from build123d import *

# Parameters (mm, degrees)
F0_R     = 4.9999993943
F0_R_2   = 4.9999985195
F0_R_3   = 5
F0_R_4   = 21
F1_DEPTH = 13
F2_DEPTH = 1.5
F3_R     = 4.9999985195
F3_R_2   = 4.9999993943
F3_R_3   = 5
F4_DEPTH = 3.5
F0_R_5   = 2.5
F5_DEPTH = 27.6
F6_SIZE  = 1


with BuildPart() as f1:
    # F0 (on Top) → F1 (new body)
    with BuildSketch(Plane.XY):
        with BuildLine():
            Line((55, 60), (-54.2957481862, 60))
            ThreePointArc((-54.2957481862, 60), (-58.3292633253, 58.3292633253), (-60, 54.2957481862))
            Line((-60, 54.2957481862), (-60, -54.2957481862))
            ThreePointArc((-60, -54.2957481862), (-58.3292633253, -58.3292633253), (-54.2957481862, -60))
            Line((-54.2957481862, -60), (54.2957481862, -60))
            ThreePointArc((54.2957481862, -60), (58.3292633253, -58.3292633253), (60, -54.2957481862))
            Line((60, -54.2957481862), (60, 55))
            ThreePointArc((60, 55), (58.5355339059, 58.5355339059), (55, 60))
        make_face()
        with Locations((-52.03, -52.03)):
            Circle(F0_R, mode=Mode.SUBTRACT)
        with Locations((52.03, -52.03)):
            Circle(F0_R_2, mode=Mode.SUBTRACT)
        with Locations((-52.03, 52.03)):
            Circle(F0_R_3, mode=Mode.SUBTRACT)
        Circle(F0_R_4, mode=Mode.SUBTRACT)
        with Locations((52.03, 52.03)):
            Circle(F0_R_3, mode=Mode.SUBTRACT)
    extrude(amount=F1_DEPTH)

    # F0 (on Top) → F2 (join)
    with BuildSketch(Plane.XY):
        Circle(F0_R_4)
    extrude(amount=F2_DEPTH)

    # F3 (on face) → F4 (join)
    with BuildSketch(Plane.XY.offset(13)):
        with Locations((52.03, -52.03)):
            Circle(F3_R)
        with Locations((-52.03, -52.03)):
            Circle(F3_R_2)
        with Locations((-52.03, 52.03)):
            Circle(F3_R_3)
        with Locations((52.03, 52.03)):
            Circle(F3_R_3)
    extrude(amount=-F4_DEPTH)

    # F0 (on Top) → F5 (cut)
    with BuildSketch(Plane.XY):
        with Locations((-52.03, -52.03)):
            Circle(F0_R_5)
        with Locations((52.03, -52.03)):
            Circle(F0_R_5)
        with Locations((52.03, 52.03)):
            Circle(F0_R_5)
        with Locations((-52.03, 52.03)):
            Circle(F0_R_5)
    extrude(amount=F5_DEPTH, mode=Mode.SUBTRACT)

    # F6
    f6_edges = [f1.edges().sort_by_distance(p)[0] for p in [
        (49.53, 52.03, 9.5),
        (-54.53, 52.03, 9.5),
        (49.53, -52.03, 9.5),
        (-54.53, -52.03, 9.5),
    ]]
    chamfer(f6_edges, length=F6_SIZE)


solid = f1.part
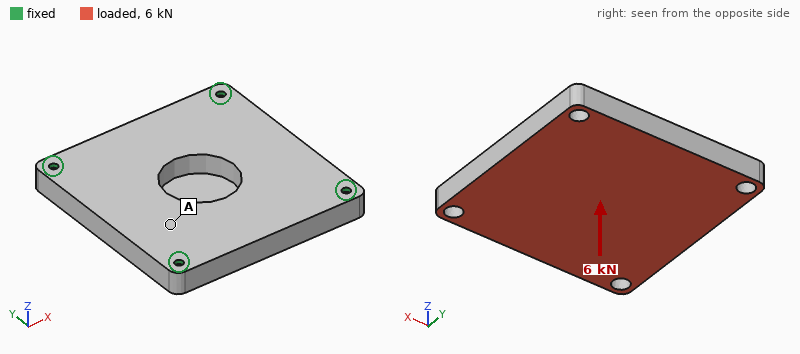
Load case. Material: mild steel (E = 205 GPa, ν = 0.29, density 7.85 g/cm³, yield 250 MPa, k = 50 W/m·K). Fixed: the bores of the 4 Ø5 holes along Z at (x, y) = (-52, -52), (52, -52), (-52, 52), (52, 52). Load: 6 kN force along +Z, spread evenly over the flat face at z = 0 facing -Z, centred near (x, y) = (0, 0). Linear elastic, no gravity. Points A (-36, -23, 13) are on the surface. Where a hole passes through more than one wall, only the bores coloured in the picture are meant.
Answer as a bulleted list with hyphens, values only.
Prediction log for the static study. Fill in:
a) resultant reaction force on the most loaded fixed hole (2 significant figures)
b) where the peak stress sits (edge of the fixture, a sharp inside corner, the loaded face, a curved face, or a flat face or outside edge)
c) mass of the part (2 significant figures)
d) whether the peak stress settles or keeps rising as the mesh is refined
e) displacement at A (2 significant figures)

- 2.7 kN
- edge of the fixture
- 1.3 kg
- keeps rising
- 15 µm
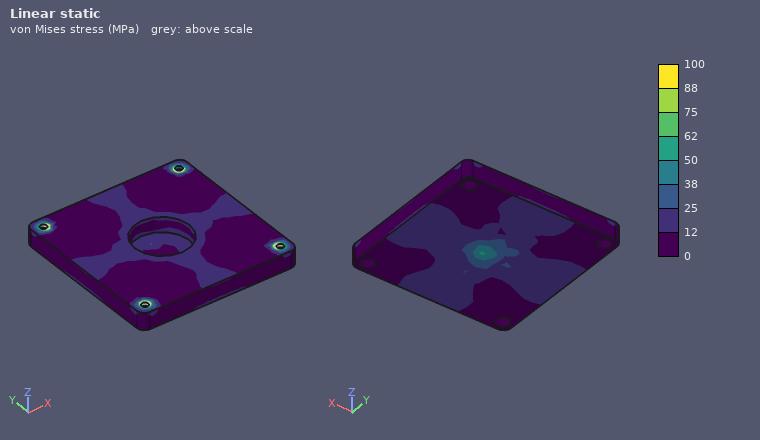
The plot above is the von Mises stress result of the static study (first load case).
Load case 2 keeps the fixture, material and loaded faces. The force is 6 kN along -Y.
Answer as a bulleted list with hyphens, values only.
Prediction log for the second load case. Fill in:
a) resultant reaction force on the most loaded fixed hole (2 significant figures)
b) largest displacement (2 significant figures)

- 1.6 kN
- 3.3 µm
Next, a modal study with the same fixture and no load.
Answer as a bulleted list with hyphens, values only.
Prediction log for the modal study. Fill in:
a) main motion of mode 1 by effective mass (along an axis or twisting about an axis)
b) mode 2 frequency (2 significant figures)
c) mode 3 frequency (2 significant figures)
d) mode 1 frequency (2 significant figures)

- along Z
- 4500 Hz
- 4500 Hz
- 2800 Hz
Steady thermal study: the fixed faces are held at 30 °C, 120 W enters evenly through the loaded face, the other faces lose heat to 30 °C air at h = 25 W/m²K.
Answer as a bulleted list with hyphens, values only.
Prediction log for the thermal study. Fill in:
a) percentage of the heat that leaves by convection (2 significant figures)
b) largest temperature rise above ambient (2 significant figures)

- 22 %
- 67 K
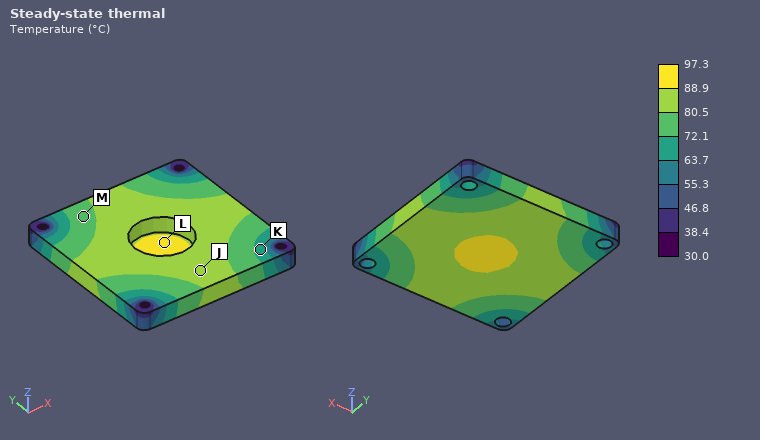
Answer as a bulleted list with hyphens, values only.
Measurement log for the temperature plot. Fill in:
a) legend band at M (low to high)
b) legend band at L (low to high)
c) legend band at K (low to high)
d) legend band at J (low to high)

- 72.1 to 80.5 °C
- 88.9 to 97.3 °C
- 63.7 to 72.1 °C
- 80.5 to 88.9 °C
